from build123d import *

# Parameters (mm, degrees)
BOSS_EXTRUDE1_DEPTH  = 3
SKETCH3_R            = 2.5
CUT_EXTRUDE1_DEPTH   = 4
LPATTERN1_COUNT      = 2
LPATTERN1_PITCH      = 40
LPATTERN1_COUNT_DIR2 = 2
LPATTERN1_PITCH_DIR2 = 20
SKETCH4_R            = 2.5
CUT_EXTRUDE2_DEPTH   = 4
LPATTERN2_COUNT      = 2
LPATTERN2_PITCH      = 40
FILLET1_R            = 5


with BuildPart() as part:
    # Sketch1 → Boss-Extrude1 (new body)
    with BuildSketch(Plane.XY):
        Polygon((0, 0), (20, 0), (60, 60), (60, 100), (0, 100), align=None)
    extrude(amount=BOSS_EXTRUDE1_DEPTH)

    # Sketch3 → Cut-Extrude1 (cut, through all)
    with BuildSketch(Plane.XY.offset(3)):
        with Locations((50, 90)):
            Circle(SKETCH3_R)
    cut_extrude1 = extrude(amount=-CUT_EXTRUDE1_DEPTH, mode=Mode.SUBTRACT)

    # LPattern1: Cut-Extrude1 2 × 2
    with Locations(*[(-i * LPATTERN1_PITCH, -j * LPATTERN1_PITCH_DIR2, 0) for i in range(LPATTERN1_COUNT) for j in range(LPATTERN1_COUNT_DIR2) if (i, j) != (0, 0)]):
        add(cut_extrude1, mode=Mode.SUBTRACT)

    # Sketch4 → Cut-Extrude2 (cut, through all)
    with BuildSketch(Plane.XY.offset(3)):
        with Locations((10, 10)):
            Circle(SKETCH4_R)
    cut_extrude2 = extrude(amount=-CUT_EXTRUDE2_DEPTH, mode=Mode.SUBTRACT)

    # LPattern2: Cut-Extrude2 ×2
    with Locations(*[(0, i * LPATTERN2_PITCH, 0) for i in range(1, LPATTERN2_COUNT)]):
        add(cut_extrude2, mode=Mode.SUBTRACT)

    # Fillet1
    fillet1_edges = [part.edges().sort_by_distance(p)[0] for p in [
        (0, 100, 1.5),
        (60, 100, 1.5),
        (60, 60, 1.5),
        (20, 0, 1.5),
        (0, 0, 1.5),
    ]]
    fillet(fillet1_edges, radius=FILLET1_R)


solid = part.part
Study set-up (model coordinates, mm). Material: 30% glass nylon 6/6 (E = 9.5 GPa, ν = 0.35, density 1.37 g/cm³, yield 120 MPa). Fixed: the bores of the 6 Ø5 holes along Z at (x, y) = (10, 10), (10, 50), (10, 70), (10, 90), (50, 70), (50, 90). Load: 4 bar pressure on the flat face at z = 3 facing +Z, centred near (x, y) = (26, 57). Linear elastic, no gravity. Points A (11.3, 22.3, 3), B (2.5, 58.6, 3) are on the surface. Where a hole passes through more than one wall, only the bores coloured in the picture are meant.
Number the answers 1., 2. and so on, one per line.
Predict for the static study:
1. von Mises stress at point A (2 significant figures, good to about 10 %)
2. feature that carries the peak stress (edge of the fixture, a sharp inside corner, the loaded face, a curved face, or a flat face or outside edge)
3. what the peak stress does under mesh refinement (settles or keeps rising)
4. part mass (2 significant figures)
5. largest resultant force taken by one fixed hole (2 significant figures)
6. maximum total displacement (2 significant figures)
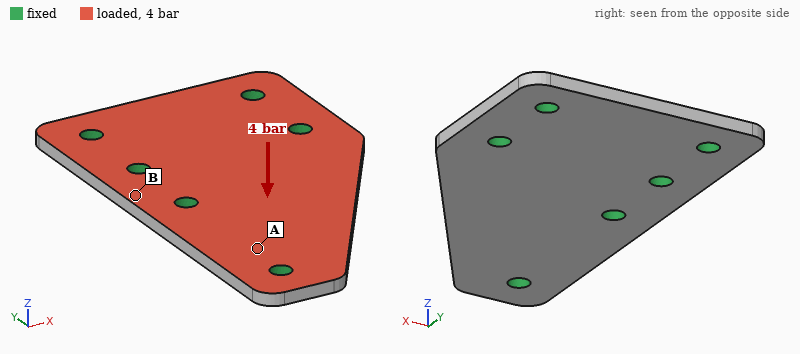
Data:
1. 27 MPa
2. edge of the fixture
3. keeps rising
4. 19 g
5. 430 N
6. 1.1 mm
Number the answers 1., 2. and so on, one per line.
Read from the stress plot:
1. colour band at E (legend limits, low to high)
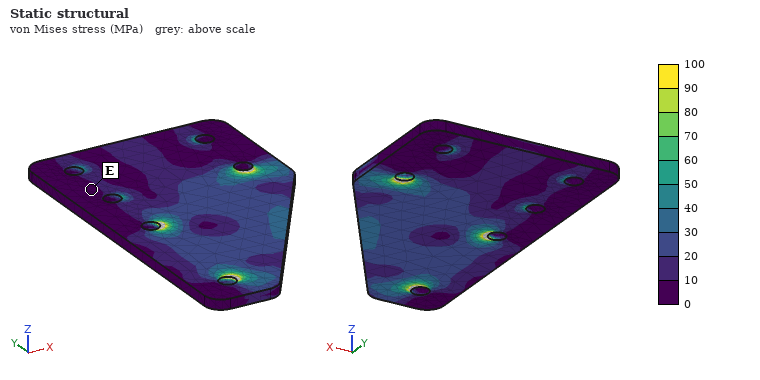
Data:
1. 0 to 10 MPa
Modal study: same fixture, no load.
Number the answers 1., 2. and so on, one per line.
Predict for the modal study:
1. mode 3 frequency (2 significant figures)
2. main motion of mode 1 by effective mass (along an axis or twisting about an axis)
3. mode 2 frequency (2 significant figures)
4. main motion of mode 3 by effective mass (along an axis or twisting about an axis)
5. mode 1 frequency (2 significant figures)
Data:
1. 5400 Hz
2. along Z
3. 4400 Hz
4. along Z
5. 2000 Hz
